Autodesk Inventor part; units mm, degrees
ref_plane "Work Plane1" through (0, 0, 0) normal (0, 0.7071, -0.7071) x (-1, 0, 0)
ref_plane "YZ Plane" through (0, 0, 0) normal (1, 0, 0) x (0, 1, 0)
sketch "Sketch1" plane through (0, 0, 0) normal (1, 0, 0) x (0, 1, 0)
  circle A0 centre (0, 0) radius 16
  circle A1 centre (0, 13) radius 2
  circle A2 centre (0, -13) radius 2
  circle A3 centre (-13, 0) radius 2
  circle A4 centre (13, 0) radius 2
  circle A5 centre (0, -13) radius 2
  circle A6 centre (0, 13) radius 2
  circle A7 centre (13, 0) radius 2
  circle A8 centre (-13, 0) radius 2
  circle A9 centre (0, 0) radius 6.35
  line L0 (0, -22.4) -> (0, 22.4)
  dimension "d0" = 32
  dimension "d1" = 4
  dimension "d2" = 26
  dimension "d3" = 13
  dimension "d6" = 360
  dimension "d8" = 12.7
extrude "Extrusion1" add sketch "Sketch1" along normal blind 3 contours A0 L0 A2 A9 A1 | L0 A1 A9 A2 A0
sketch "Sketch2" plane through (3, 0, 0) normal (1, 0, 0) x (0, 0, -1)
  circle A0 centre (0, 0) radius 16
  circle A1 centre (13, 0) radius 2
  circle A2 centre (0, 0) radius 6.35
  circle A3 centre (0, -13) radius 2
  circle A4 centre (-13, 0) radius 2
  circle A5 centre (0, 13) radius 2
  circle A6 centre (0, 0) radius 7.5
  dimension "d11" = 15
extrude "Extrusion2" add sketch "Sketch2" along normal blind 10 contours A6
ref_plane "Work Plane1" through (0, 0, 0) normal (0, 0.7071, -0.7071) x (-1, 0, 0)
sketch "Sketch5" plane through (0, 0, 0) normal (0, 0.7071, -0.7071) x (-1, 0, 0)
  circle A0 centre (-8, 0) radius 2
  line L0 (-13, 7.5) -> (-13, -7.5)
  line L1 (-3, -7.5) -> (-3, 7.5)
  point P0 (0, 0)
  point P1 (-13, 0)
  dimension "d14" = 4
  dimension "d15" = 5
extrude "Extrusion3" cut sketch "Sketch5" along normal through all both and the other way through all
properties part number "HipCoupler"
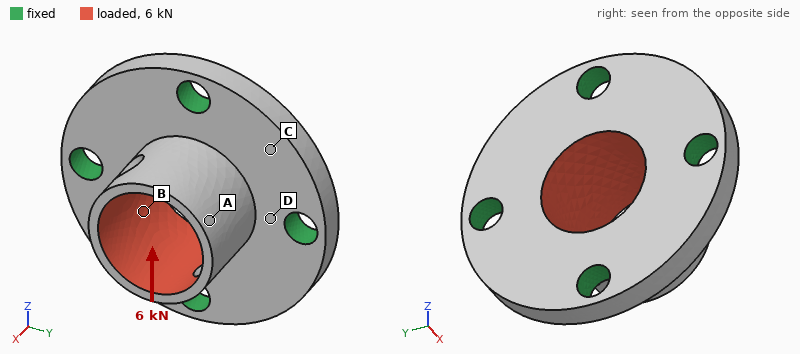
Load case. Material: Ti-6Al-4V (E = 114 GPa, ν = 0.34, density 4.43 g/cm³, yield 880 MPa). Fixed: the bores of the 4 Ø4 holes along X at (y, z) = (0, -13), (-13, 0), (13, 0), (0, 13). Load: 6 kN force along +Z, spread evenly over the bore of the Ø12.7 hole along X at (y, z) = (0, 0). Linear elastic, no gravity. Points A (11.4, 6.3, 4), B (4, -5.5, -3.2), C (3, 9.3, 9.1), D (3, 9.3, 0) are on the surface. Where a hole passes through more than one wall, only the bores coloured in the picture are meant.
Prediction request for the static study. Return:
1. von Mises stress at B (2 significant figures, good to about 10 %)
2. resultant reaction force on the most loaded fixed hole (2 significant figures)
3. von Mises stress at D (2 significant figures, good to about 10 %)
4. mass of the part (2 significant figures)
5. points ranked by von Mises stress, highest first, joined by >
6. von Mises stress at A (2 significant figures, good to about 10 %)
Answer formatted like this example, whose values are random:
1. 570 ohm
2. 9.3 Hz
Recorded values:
1. 230 MPa
2. 2.2 kN
3. 140 MPa
4. 10 g
5. B > D > A > C
6. 67 MPa
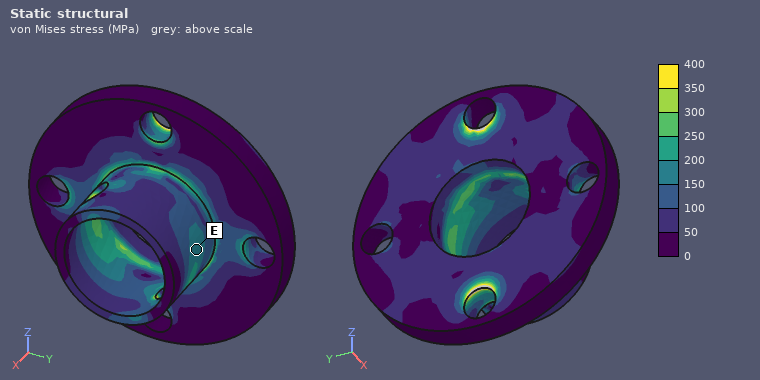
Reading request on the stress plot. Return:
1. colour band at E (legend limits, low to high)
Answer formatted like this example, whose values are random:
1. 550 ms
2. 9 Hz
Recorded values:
1. 150 to 200 MPa
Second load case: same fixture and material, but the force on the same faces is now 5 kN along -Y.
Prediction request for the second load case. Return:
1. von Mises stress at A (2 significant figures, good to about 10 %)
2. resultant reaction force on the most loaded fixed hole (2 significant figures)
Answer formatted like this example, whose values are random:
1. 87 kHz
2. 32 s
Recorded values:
1. 62 MPa
2. 1.9 kN
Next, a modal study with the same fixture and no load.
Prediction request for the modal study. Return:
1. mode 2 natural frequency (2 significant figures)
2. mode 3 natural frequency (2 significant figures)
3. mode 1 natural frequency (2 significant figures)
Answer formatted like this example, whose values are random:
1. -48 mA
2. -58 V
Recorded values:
1. 28 kHz
2. 30 kHz
3. 26 kHz
